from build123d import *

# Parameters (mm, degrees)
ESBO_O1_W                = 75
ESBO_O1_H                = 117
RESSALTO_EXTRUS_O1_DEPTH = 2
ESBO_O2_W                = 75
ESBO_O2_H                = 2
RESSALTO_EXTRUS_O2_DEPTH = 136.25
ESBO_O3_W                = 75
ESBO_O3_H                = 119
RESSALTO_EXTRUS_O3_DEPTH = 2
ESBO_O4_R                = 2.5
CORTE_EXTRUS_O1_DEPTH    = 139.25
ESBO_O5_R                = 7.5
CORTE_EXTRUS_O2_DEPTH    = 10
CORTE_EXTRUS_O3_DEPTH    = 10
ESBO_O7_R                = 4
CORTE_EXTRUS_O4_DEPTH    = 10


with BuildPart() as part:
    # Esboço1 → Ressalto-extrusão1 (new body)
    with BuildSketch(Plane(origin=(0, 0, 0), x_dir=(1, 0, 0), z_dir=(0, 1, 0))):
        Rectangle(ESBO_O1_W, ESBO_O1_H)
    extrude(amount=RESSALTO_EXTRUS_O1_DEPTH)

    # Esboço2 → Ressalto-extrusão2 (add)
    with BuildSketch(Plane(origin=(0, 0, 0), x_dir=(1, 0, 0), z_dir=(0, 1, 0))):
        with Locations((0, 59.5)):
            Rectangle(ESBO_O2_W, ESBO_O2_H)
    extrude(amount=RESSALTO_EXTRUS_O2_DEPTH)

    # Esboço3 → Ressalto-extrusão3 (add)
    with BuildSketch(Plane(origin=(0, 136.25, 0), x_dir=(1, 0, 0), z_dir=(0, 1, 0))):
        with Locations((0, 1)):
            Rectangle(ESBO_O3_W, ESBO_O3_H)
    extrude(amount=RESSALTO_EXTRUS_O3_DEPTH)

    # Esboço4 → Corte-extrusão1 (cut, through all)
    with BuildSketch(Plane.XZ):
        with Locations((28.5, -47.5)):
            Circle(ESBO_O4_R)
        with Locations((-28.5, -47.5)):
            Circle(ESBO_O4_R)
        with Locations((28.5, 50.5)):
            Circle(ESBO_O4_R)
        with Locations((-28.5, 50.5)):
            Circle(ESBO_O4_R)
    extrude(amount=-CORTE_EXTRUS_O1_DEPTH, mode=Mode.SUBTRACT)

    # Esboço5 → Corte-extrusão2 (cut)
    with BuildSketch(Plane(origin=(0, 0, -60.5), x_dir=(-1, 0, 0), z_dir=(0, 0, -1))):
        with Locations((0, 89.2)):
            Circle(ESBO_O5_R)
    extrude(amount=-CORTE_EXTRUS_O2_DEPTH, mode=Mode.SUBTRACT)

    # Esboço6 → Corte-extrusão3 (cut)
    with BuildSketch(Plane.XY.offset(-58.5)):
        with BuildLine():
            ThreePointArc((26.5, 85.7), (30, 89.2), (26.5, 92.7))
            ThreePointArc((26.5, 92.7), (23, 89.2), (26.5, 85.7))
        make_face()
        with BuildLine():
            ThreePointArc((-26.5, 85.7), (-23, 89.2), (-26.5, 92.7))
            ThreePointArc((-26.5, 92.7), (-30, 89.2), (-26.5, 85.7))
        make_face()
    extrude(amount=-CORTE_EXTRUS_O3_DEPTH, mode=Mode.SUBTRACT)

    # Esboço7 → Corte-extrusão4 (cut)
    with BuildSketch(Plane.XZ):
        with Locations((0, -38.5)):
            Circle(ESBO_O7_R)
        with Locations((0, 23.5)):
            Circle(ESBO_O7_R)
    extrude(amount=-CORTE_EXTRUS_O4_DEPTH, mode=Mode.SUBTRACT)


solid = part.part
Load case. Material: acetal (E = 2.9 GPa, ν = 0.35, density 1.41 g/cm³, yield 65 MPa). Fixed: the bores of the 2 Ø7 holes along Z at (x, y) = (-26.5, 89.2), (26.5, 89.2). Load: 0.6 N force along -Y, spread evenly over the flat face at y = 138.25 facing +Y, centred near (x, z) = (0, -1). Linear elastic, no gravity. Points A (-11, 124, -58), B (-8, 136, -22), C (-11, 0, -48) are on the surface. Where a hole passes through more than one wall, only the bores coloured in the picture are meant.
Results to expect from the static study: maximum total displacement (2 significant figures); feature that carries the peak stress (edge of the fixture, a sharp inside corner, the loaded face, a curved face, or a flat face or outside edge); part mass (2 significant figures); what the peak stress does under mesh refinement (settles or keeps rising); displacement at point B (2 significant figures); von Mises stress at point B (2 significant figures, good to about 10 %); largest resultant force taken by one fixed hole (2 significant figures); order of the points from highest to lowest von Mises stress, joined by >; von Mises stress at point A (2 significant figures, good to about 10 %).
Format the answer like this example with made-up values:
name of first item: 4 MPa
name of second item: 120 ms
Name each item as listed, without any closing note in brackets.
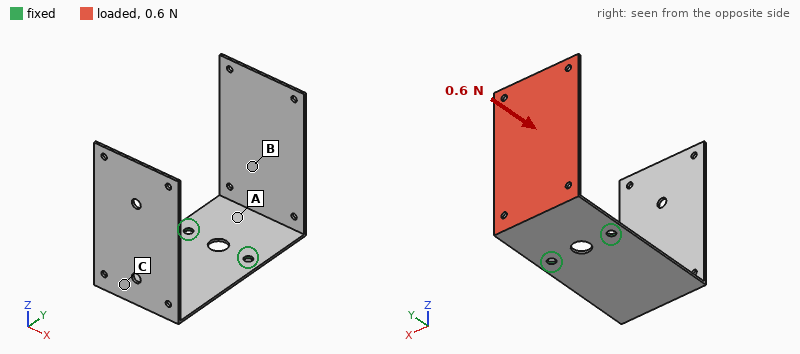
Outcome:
maximum total displacement: 2.1 mm
feature that carries the peak stress: edge of the fixture
part mass: 77 g
what the peak stress does under mesh refinement: keeps rising
displacement at point B: 0.58 mm
von Mises stress at point B: 0.30 MPa
largest resultant force taken by one fixed hole: 0.32 N
order of the points from highest to lowest von Mises stress, joined by >: A > B > C
von Mises stress at point A: 0.64 MPa
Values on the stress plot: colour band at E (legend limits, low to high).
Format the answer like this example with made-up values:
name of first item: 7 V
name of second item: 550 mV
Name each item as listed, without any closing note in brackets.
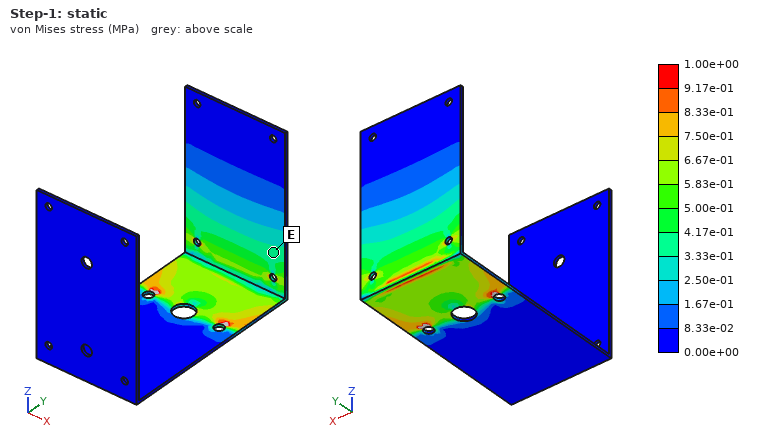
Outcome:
colour band at E: 3.33e-01 to 4.17e-01 MPa
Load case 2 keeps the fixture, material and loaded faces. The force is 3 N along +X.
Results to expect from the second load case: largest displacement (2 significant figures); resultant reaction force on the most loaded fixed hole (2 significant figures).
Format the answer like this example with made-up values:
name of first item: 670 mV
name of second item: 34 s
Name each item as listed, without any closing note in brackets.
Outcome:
largest displacement: 2.2 mm
resultant reaction force on the most loaded fixed hole: 4.3 N
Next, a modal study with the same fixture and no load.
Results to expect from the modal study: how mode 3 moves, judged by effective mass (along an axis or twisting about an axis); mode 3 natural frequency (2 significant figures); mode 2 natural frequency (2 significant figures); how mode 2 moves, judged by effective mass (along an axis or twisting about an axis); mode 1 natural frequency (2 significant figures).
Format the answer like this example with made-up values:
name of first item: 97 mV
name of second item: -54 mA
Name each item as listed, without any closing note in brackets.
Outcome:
how mode 3 moves, judged by effective mass: along X
mode 3 natural frequency: 27 Hz
mode 2 natural frequency: 21 Hz
how mode 2 moves, judged by effective mass: along Y
mode 1 natural frequency: 15 Hz
